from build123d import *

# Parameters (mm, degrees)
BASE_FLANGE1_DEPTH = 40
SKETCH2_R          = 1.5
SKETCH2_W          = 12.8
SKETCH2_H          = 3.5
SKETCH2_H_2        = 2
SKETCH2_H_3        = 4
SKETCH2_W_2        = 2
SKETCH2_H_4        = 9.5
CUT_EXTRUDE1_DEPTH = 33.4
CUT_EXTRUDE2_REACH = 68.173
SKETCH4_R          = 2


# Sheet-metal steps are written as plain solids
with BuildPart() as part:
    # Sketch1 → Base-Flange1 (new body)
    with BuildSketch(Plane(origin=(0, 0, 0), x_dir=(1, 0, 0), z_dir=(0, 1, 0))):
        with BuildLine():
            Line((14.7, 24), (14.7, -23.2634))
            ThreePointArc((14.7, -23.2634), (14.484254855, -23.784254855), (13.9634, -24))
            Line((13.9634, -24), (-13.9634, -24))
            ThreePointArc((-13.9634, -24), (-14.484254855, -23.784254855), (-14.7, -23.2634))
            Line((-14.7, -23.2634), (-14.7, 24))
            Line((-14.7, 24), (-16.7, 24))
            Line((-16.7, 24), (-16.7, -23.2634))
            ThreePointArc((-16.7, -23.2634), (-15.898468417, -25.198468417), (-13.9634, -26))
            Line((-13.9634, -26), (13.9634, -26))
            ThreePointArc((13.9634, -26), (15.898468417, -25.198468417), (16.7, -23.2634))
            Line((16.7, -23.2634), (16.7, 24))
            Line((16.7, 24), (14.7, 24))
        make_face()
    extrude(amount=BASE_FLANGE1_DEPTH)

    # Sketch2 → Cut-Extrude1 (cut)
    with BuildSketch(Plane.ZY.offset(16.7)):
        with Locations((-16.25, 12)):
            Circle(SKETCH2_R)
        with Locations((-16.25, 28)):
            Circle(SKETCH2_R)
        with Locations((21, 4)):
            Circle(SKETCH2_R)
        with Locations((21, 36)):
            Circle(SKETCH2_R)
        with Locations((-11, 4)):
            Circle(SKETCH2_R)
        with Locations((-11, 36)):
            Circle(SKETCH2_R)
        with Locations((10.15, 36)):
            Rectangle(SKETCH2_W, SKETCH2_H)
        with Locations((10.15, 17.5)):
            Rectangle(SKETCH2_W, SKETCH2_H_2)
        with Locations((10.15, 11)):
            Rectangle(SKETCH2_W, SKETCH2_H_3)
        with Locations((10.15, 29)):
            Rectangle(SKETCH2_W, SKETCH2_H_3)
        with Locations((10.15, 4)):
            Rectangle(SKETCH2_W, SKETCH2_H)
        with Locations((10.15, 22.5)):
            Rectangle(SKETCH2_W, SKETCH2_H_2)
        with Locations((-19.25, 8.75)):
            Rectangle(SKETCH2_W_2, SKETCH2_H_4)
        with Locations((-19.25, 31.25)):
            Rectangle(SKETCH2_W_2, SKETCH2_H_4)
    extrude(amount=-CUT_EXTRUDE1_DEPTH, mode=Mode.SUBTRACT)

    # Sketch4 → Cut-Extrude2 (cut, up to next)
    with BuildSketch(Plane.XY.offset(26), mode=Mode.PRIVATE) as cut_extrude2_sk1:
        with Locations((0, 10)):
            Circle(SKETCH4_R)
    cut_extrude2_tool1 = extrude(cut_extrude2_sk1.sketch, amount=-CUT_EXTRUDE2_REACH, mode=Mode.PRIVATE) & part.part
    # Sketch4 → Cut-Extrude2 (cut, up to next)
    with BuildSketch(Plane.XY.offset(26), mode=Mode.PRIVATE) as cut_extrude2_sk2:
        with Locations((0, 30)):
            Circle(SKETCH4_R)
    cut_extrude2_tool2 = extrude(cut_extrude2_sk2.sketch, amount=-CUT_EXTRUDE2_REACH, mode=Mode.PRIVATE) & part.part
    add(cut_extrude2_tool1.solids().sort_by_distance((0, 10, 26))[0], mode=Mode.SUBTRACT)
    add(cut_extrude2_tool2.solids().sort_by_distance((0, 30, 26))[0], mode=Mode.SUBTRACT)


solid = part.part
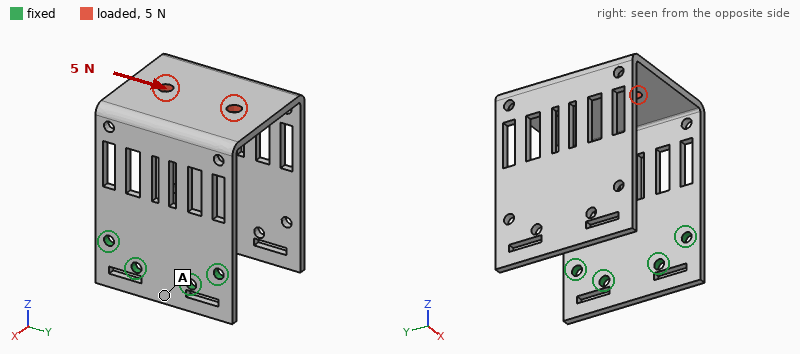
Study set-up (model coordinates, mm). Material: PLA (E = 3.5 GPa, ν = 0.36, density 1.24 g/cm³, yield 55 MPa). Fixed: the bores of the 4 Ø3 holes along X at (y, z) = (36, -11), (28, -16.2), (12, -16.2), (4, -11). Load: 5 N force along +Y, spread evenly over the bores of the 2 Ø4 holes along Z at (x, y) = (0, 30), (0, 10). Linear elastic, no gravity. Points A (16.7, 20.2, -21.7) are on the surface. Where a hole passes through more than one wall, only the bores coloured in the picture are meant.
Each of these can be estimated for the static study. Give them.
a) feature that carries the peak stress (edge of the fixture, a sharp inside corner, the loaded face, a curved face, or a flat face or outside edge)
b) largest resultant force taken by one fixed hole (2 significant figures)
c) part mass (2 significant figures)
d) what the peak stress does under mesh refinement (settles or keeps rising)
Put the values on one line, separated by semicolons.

edge of the fixture; 6.2 N; 11 g; keeps rising
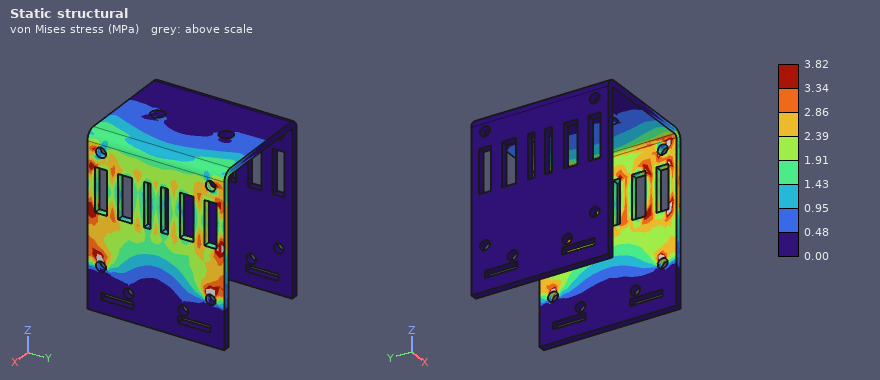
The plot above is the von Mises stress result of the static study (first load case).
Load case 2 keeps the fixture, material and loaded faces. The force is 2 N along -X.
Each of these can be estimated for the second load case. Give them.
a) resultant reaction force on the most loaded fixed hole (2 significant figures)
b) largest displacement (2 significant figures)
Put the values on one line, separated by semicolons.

1.9 N; 0.75 mm
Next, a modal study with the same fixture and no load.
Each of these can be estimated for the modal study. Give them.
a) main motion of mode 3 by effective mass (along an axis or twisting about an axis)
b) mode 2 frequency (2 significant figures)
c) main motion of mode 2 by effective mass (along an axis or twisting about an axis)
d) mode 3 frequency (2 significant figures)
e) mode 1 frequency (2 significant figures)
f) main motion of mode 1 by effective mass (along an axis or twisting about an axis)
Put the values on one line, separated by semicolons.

along X; 110 Hz; along Y; 140 Hz; 73 Hz; along Z
